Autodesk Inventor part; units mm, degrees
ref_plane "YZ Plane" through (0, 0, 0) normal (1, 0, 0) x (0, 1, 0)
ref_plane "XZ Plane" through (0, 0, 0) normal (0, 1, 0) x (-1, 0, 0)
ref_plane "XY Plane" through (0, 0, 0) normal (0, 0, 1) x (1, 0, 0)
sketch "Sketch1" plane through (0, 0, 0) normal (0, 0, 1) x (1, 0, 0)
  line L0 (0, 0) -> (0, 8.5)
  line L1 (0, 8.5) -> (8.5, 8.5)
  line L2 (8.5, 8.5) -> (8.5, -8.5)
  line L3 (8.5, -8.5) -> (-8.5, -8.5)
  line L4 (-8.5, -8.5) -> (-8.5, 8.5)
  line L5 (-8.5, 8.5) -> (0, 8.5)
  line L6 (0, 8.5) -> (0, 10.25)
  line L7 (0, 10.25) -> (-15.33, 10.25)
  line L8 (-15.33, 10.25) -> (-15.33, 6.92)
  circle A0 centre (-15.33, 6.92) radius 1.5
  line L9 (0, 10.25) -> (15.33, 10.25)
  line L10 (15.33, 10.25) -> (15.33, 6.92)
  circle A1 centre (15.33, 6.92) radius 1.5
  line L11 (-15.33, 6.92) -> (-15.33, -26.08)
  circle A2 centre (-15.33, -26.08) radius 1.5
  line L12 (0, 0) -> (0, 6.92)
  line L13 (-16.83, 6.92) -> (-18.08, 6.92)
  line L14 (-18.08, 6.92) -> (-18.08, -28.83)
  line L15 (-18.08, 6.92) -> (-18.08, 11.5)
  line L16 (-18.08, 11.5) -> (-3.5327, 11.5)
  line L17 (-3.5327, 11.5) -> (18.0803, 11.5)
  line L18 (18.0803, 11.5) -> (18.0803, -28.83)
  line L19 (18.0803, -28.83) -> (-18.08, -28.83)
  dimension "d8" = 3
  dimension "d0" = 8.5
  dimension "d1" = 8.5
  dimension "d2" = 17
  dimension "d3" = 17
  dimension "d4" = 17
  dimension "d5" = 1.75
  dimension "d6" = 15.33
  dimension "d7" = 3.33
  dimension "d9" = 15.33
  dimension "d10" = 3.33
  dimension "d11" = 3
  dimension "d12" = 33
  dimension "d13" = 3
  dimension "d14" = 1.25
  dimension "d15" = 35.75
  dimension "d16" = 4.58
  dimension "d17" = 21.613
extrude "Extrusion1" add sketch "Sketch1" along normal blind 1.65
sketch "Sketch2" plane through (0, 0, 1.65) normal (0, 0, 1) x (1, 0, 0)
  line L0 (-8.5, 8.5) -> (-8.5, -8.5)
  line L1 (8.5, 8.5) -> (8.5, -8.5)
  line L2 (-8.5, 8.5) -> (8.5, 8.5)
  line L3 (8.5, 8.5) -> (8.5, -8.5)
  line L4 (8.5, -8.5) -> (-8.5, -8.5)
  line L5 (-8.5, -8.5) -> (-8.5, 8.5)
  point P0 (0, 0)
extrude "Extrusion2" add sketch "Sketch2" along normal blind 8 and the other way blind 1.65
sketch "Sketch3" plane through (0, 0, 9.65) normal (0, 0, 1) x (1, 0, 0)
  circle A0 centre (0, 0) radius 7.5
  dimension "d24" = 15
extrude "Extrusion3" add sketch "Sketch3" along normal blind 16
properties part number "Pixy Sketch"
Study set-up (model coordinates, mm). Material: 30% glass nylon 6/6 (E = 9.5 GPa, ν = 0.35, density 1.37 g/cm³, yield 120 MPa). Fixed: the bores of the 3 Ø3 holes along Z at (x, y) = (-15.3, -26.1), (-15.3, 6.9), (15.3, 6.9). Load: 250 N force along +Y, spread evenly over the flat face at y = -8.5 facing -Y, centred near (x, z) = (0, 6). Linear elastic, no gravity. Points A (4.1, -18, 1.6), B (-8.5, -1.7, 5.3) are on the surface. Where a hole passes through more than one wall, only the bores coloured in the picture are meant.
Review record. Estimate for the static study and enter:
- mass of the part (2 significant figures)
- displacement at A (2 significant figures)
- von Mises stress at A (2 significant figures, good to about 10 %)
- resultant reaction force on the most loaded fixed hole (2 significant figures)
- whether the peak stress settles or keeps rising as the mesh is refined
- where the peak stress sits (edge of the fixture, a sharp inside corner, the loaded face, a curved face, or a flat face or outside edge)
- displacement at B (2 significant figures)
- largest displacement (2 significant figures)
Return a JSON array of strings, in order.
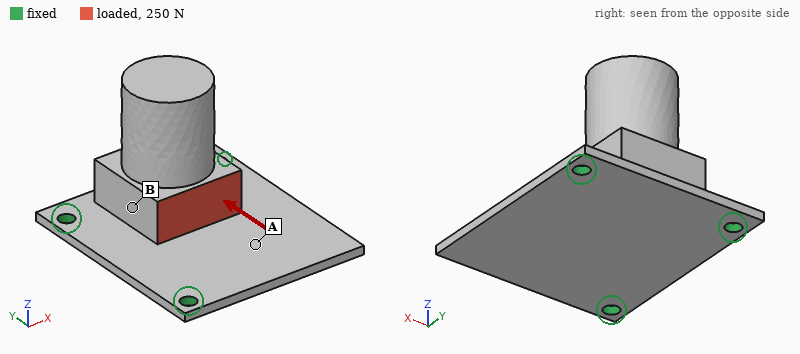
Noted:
["10 g", "0.26 mm", "11 MPa", "110 N", "keeps rising", "edge of the fixture", "0.12 mm", "0.43 mm"]
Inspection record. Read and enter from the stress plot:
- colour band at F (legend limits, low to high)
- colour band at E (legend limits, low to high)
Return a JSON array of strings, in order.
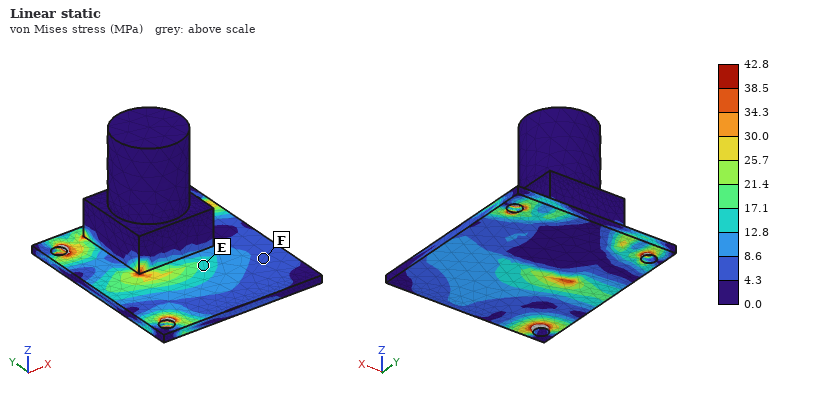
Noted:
["4.3 to 8.6 MPa", "12.8 to 17.1 MPa"]
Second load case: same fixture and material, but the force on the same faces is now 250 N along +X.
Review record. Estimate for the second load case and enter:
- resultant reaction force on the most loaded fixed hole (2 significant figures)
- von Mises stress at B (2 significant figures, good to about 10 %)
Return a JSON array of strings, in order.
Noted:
["130 N", "2.9 MPa"]
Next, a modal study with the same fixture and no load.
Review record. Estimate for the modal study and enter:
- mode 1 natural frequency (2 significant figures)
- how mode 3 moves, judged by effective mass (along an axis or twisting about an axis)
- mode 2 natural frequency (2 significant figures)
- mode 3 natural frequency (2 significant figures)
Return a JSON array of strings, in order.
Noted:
["960 Hz", "along X", "2000 Hz", "2400 Hz"]
